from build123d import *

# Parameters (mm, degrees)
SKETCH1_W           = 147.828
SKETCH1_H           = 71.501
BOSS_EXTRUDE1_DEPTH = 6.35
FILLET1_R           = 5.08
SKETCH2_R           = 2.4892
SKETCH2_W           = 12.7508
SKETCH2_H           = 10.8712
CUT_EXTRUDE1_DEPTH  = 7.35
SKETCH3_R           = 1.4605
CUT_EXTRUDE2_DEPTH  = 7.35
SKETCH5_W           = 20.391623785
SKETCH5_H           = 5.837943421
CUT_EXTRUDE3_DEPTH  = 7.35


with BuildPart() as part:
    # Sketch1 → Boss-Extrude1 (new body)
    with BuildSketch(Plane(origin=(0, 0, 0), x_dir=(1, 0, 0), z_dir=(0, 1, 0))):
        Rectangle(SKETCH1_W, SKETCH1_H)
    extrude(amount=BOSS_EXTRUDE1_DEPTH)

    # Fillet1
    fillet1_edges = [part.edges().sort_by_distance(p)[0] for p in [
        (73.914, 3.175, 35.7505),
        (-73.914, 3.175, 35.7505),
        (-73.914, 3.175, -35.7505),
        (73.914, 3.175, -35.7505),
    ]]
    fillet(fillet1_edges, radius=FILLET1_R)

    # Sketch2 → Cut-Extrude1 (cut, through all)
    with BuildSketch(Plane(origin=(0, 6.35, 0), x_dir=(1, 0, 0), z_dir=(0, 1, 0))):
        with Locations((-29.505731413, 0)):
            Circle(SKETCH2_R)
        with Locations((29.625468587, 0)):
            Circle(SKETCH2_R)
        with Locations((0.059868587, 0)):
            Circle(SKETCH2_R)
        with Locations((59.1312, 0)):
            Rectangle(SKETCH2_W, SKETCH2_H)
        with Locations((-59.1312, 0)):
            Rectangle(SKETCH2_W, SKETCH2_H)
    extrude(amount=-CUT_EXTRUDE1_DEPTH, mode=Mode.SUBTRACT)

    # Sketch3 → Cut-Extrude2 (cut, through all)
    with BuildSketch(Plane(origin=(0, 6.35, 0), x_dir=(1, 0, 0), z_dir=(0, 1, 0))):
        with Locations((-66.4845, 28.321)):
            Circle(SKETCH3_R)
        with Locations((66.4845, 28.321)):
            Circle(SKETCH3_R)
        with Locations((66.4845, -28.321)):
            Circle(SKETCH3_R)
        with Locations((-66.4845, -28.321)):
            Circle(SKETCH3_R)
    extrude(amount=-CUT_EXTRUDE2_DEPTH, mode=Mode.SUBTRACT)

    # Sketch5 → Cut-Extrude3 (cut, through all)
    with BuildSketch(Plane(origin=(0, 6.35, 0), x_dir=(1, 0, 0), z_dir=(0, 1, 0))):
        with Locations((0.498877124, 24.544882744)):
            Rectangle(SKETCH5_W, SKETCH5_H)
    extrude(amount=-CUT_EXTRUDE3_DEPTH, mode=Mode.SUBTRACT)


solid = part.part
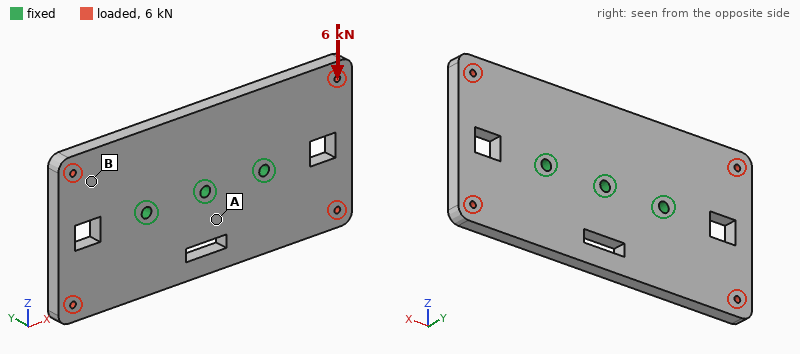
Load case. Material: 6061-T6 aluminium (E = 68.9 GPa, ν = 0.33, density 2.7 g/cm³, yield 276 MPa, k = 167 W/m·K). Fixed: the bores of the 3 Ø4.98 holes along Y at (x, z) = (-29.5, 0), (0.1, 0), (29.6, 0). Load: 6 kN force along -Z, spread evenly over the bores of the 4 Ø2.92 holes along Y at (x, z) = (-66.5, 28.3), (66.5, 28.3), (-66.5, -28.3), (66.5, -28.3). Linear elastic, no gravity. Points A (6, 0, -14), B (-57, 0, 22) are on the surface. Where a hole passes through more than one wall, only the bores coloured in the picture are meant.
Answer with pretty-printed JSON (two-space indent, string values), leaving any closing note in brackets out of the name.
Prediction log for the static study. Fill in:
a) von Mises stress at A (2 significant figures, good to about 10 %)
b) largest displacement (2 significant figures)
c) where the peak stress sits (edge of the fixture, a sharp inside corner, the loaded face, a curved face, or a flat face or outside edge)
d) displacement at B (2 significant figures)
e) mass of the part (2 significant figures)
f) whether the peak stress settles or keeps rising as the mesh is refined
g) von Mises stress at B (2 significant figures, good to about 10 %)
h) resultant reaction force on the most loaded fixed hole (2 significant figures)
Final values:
{
  "von Mises stress at A": "7.0 MPa",
  "largest displacement": "39 µm",
  "where the peak stress sits": "edge of the fixture",
  "displacement at B": "23 µm",
  "mass of the part": "170 g",
  "whether the peak stress settles or keeps rising as the mesh is refined": "keeps rising",
  "von Mises stress at B": "17 MPa",
  "resultant reaction force on the most loaded fixed hole": "3.4 kN"
}
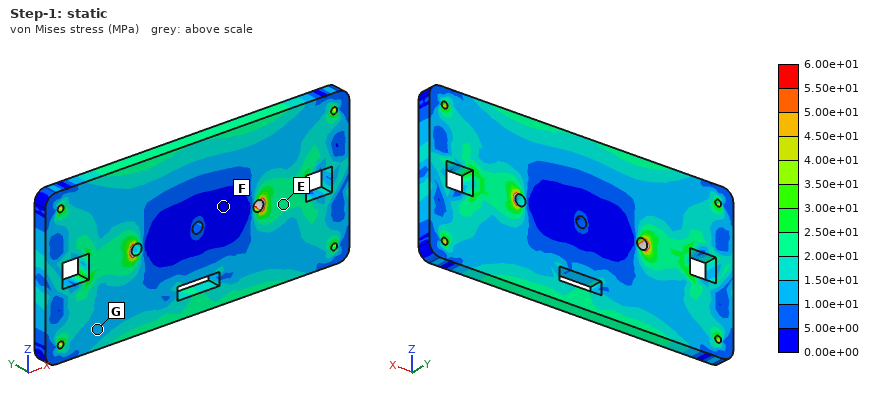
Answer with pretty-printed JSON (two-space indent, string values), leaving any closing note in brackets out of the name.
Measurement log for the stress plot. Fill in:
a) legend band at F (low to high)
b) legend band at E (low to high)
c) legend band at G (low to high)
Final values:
{
  "legend band at F": "0.00e+00 to 5.00e+00 MPa",
  "legend band at E": "2.00e+01 to 2.50e+01 MPa",
  "legend band at G": "1.00e+01 to 1.50e+01 MPa"
}
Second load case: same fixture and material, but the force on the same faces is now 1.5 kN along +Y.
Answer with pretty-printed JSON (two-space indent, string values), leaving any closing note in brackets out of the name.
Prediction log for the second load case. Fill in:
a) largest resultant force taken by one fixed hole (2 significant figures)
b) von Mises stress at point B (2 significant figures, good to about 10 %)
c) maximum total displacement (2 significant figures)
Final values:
{
  "largest resultant force taken by one fixed hole": "1.2 kN",
  "von Mises stress at point B": "16 MPa",
  "maximum total displacement": "0.25 mm"
}
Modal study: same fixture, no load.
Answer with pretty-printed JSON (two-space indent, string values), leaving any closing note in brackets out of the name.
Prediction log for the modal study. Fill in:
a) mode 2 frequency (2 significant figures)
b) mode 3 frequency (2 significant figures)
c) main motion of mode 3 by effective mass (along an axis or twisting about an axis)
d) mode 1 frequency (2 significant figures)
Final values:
{
  "mode 2 frequency": "2200 Hz",
  "mode 3 frequency": "2300 Hz",
  "main motion of mode 3 by effective mass": "twisting about X",
  "mode 1 frequency": "2200 Hz"
}
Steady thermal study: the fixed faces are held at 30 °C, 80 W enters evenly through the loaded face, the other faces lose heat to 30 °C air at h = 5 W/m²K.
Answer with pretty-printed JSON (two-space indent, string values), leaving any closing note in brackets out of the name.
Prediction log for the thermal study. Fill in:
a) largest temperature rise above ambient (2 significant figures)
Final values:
{
  "largest temperature rise above ambient": "36 K"
}
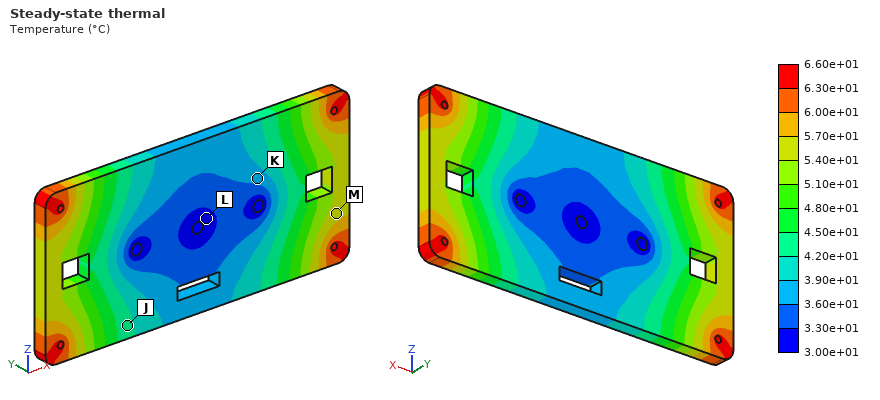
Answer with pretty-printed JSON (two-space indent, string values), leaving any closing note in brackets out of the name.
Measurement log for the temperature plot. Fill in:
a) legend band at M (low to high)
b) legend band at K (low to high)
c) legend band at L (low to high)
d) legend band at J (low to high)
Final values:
{
  "legend band at M": "5.40e+01 to 5.70e+01 °C",
  "legend band at K": "3.60e+01 to 3.90e+01 °C",
  "legend band at L": "3.00e+01 to 3.30e+01 °C",
  "legend band at J": "4.20e+01 to 4.50e+01 °C"
}
